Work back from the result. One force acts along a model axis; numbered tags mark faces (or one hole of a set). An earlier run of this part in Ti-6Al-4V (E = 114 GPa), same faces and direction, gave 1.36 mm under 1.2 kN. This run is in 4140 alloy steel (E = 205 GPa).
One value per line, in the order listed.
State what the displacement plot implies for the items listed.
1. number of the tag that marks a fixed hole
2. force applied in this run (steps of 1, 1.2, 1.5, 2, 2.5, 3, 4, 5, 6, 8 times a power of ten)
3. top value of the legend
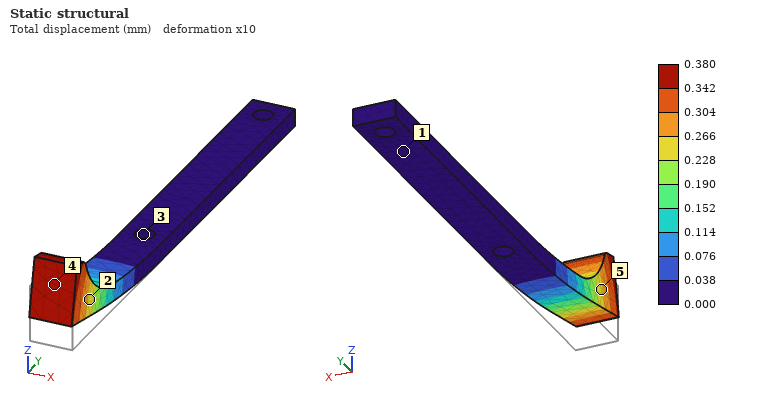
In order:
3
600 N
0.380 mm
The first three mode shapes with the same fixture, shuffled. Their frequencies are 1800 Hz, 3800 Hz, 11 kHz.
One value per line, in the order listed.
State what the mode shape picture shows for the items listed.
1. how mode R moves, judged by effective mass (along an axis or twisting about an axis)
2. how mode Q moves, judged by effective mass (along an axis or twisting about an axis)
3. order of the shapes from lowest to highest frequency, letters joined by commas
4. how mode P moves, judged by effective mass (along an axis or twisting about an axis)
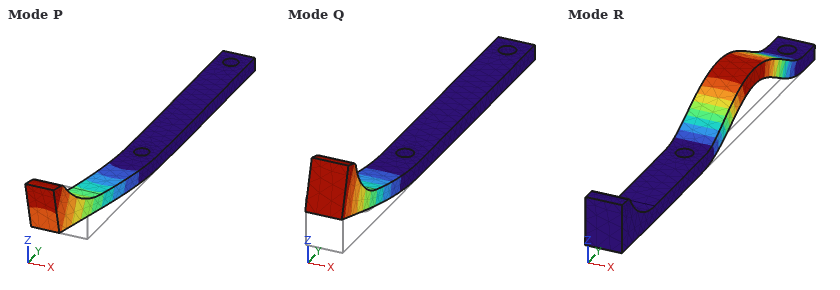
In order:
along Z
along Z
Q, P, R
along X
